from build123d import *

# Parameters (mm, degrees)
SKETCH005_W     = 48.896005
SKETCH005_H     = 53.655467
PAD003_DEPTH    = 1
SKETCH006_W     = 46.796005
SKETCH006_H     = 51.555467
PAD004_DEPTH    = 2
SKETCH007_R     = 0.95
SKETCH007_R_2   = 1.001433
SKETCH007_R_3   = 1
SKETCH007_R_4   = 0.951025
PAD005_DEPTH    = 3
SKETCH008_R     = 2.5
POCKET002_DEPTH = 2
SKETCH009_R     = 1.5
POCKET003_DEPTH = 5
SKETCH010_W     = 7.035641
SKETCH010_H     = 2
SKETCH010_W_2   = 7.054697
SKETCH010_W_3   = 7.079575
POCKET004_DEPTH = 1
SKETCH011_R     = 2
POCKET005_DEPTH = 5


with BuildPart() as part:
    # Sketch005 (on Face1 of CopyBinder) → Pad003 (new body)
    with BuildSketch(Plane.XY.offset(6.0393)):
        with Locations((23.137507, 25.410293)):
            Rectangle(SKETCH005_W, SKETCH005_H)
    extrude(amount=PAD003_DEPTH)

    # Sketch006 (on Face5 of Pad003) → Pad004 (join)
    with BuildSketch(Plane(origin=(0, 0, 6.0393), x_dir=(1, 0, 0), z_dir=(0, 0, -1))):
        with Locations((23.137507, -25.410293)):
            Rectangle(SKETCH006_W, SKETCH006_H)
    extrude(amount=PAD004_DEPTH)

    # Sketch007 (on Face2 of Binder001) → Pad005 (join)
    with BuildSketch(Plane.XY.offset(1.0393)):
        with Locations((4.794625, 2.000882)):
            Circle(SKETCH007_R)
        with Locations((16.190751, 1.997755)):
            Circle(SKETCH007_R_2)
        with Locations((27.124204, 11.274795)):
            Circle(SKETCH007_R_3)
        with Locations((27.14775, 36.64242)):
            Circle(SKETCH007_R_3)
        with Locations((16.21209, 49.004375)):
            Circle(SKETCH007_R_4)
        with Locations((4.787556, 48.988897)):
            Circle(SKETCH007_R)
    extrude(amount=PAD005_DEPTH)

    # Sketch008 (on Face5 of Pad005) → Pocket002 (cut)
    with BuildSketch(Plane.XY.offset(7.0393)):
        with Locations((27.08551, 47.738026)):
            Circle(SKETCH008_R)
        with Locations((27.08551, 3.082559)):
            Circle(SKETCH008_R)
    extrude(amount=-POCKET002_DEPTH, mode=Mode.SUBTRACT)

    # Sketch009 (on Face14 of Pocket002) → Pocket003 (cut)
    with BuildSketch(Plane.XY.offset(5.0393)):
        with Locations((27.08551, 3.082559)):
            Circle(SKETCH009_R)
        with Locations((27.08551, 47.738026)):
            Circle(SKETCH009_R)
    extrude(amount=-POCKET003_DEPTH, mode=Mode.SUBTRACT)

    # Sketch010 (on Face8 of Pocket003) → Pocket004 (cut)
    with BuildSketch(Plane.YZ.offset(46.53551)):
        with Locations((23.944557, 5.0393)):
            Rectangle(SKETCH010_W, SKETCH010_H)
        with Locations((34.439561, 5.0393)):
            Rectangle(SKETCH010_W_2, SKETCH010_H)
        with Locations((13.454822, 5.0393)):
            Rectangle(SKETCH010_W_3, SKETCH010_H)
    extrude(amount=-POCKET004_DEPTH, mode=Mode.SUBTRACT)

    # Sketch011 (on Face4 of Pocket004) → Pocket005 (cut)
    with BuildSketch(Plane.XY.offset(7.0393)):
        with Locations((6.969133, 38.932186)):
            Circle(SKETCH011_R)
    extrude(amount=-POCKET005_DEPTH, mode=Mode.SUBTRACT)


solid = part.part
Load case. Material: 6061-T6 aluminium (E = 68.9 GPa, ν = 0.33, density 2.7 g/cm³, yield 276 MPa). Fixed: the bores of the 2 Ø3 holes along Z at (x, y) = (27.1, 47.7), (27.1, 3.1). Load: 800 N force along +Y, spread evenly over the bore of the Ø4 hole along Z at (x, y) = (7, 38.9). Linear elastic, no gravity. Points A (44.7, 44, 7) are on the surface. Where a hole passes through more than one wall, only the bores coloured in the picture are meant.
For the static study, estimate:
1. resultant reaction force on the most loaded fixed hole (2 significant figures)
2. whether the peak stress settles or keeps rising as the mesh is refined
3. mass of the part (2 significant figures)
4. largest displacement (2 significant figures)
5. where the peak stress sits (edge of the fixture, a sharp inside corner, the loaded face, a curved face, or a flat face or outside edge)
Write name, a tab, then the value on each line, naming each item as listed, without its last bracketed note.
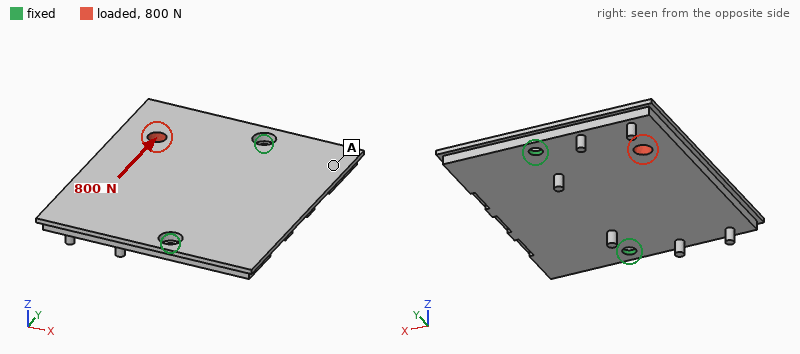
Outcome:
resultant reaction force on the most loaded fixed hole	540 N
whether the peak stress settles or keeps rising as the mesh is refined	keeps rising
mass of the part	20 g
largest displacement	20 µm
where the peak stress sits	edge of the fixture
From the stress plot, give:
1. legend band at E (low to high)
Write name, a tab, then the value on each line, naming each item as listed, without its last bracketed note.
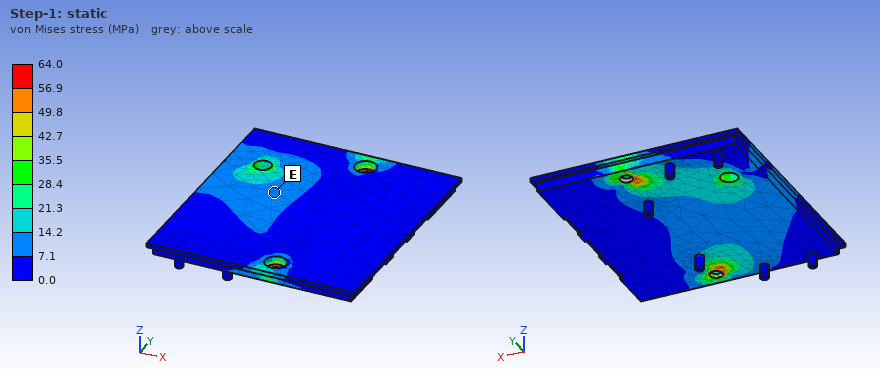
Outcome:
legend band at E	7.1 to 14.2 MPa
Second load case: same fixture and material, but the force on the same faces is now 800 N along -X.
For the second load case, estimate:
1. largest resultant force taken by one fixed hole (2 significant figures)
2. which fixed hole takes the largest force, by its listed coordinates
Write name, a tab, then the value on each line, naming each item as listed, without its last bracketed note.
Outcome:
largest resultant force taken by one fixed hole	640 N
which fixed hole takes the largest force, by its listed coordinates	(27.1, 47.7)
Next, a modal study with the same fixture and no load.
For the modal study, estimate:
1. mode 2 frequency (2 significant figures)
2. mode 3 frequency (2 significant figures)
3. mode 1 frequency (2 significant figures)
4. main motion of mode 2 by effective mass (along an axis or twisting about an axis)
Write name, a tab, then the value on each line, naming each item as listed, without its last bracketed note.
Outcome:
mode 2 frequency	3600 Hz
mode 3 frequency	4100 Hz
mode 1 frequency	1400 Hz
main motion of mode 2 by effective mass	along Z
